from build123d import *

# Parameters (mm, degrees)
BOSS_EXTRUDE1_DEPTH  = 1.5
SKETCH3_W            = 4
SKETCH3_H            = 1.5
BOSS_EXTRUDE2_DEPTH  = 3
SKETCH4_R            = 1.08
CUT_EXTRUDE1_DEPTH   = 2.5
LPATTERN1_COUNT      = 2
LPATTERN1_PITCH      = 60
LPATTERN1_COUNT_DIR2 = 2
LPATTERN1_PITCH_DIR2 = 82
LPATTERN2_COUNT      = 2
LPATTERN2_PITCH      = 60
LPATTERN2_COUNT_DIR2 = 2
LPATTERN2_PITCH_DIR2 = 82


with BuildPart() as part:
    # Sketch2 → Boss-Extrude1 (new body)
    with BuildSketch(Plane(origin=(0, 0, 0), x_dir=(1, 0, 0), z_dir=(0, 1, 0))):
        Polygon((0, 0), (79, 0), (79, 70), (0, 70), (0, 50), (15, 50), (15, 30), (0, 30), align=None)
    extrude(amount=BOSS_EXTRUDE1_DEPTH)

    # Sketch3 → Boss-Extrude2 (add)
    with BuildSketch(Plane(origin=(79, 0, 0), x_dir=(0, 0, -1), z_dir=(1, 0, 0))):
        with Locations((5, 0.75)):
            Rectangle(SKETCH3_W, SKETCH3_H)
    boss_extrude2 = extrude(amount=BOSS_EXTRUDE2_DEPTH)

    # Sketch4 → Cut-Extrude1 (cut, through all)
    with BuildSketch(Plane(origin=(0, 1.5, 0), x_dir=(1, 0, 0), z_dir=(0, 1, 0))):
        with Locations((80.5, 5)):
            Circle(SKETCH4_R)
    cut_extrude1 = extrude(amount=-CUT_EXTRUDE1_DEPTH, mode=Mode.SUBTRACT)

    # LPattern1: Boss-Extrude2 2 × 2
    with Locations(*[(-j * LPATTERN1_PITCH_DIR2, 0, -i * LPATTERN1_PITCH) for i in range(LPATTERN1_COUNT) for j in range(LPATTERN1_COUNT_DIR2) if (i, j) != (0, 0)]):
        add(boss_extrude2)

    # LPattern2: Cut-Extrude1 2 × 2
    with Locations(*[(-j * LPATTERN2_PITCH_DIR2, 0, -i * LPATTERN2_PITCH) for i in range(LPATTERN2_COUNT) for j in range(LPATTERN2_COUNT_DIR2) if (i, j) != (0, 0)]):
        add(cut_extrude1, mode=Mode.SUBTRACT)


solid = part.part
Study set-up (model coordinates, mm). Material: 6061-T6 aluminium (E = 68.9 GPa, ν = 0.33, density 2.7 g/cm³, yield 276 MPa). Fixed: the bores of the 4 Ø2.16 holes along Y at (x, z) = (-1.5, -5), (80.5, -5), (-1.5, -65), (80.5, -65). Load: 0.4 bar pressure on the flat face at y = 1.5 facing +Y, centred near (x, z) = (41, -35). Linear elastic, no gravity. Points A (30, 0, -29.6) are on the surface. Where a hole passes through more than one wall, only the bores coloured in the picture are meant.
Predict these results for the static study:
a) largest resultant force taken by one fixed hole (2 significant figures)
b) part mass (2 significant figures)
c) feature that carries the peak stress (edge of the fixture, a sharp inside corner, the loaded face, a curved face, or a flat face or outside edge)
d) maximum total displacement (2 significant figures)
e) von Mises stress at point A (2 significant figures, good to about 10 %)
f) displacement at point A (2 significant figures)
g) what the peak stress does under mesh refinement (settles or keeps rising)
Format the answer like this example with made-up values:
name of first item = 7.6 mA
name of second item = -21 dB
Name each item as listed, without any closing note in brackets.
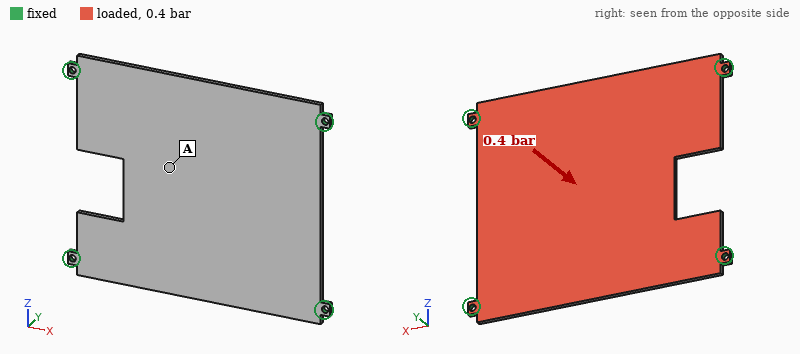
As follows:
largest resultant force taken by one fixed hole = 55 N
part mass = 21 g
feature that carries the peak stress = edge of the fixture
maximum total displacement = 0.58 mm
von Mises stress at point A = 36 MPa
displacement at point A = 0.55 mm
what the peak stress does under mesh refinement = keeps rising
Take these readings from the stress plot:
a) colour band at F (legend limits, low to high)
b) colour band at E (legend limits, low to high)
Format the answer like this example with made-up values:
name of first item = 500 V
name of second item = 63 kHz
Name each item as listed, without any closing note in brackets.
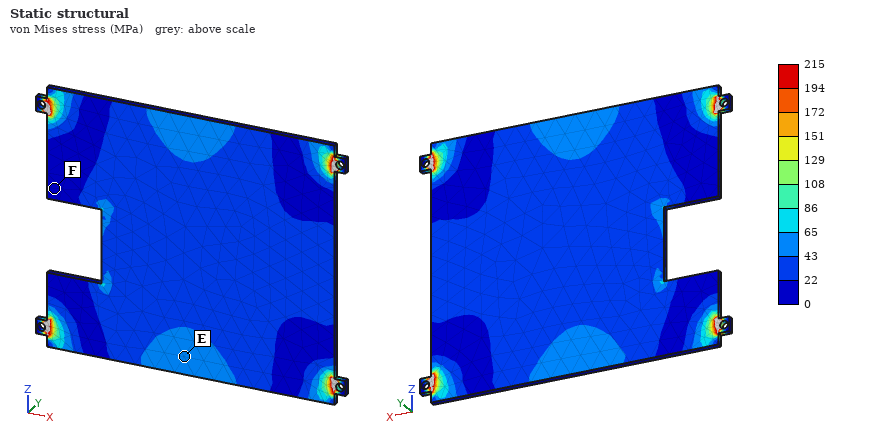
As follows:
colour band at F = 0 to 22 MPa
colour band at E = 43 to 65 MPa
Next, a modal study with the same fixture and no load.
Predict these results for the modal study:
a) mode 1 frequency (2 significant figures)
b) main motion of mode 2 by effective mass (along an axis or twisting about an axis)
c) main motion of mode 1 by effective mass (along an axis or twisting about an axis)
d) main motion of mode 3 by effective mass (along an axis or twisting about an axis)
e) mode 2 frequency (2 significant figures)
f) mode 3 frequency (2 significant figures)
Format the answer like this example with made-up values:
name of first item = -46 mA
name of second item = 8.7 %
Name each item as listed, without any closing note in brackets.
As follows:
mode 1 frequency = 760 Hz
main motion of mode 2 by effective mass = twisting about X
main motion of mode 1 by effective mass = along Y
main motion of mode 3 by effective mass = twisting about Z
mode 2 frequency = 1300 Hz
mode 3 frequency = 1800 Hz
